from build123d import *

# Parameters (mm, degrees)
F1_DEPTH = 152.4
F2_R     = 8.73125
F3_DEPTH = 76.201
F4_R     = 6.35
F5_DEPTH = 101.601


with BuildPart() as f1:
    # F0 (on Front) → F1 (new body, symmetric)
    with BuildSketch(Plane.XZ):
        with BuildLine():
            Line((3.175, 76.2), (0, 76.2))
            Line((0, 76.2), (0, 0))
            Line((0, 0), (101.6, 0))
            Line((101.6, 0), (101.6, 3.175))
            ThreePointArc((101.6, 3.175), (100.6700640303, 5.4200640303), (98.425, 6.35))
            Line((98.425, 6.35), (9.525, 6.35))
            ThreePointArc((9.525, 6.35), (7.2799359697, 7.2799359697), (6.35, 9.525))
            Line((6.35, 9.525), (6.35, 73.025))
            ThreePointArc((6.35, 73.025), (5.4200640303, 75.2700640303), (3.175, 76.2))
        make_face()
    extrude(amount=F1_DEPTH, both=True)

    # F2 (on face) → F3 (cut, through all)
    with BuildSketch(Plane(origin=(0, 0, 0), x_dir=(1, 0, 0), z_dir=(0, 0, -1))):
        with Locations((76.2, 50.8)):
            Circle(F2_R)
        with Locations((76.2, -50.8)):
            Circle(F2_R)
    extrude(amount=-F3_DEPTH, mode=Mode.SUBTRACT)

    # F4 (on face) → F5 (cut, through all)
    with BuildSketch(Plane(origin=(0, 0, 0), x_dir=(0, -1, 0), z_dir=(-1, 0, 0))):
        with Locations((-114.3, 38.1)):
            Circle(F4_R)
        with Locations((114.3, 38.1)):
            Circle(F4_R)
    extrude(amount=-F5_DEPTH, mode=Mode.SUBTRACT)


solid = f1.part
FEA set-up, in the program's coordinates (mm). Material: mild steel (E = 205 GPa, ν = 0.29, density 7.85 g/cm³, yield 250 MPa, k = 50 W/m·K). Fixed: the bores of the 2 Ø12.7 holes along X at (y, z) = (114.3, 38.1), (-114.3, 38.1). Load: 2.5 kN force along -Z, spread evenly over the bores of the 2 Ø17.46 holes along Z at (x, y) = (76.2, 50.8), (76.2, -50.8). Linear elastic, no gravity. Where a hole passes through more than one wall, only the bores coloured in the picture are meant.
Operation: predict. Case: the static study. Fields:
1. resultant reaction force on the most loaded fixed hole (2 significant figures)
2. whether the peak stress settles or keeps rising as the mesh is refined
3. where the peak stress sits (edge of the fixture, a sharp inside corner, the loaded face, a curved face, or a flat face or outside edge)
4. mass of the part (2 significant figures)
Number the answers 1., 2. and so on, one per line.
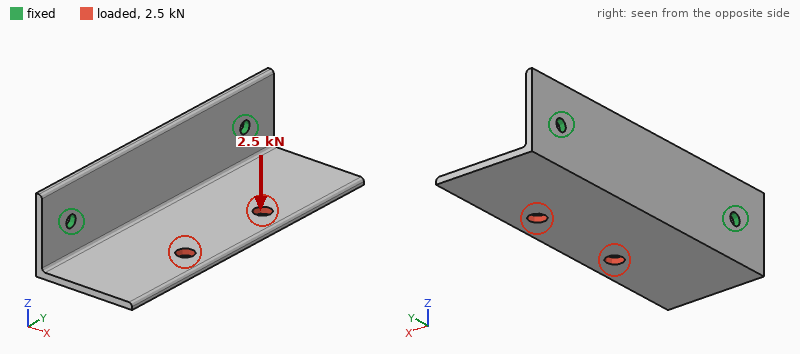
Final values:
1. 1.3 kN
2. keeps rising
3. edge of the fixture
4. 2.6 kg
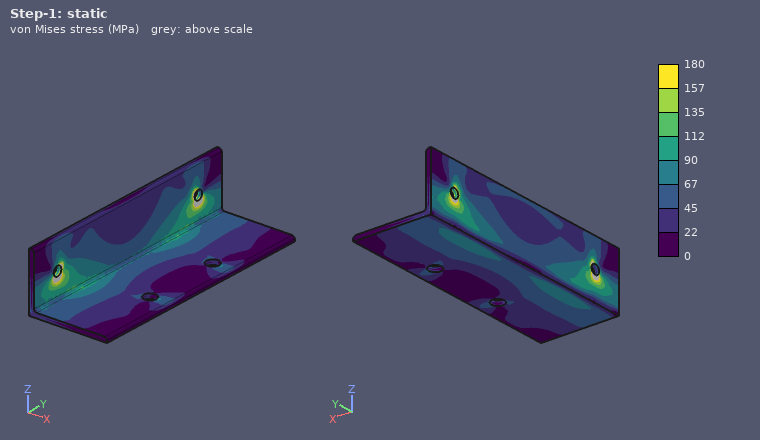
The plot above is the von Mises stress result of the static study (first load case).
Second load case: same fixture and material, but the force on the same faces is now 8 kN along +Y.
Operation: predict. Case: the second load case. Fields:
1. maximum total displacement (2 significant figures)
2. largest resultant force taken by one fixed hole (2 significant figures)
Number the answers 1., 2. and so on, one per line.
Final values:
1. 0.26 mm
2. 4.9 kN
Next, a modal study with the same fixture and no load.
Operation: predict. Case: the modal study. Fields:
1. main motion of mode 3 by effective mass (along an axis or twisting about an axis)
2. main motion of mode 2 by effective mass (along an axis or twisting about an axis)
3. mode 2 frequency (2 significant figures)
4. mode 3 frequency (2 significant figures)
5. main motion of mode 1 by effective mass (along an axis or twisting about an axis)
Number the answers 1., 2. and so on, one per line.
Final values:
1. along X
2. twisting about X
3. 510 Hz
4. 840 Hz
5. along Z
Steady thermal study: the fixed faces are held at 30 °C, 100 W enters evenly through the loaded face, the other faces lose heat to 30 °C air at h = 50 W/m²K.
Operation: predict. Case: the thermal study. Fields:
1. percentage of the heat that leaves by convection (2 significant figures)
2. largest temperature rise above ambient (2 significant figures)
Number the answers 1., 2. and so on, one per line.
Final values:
1. 91 %
2. 78 K
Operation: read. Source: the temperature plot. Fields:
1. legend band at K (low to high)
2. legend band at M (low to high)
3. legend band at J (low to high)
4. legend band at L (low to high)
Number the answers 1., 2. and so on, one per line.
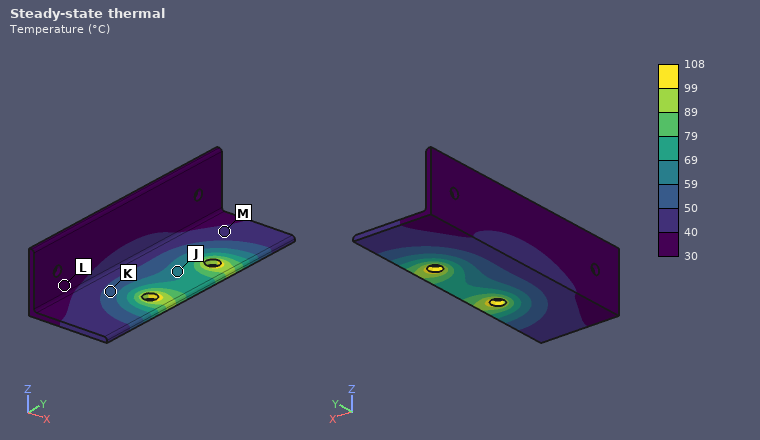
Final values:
1. 50 to 59 °C
2. 40 to 50 °C
3. 59 to 69 °C
4. 30 to 40 °C
